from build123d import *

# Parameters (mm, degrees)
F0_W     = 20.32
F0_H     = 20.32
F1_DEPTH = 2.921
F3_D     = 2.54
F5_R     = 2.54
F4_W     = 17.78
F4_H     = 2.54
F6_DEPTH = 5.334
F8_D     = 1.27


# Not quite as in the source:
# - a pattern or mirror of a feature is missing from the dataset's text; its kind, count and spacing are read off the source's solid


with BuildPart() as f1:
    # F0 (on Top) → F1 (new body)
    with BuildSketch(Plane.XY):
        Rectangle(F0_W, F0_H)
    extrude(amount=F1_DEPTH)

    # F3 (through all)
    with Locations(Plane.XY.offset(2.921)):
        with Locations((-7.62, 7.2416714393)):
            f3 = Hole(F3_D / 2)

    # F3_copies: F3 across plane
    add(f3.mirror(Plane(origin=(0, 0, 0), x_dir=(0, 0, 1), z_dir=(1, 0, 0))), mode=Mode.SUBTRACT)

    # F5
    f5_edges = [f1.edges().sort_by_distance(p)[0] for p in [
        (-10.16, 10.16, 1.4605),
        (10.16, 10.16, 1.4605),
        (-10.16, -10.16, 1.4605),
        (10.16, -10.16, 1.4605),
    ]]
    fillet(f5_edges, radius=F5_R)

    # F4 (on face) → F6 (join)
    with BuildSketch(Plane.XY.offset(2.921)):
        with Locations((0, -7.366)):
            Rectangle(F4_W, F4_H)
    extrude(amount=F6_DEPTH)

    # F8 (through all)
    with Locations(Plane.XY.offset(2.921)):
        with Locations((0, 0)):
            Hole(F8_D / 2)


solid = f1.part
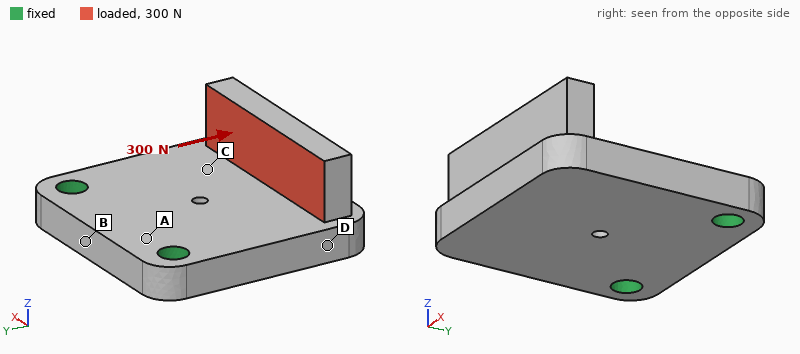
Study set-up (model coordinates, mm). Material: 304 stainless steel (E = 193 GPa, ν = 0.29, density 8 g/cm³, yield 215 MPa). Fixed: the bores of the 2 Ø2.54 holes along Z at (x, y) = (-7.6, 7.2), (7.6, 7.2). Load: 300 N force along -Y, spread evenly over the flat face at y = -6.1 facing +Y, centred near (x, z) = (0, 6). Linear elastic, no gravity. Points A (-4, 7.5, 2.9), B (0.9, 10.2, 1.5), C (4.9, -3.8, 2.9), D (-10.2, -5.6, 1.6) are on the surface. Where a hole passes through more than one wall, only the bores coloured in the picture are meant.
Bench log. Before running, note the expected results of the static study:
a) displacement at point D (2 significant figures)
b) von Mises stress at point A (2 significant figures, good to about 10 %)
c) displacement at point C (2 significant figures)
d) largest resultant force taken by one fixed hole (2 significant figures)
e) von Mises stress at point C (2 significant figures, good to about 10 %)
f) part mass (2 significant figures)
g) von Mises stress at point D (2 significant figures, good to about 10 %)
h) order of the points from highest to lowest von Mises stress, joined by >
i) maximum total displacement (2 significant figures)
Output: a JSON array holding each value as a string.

["13 µm", "24 MPa", "10 µm", "150 N", "45 MPa", "11 g", "14 MPa", "C > A > D > B", "27 µm"]
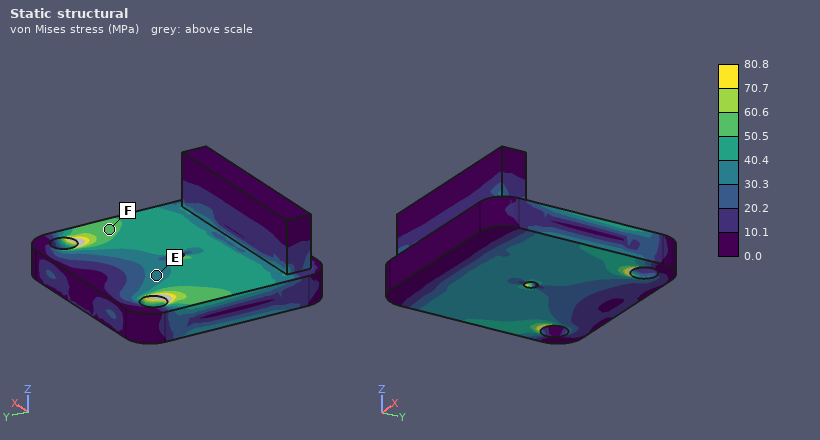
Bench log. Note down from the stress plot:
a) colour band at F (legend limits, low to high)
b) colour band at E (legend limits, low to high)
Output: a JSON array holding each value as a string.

["50.5 to 60.6 MPa", "30.3 to 40.4 MPa"]
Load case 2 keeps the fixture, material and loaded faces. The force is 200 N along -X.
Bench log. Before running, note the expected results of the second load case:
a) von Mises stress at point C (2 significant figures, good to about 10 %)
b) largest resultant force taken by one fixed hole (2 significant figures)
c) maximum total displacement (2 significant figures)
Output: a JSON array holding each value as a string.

["25 MPa", "200 N", "7.5 µm"]
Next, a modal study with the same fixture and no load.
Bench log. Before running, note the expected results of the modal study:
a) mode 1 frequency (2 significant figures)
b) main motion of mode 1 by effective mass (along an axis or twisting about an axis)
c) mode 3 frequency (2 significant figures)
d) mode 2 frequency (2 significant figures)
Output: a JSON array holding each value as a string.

["5700 Hz", "along Z", "26 kHz", "13 kHz"]
